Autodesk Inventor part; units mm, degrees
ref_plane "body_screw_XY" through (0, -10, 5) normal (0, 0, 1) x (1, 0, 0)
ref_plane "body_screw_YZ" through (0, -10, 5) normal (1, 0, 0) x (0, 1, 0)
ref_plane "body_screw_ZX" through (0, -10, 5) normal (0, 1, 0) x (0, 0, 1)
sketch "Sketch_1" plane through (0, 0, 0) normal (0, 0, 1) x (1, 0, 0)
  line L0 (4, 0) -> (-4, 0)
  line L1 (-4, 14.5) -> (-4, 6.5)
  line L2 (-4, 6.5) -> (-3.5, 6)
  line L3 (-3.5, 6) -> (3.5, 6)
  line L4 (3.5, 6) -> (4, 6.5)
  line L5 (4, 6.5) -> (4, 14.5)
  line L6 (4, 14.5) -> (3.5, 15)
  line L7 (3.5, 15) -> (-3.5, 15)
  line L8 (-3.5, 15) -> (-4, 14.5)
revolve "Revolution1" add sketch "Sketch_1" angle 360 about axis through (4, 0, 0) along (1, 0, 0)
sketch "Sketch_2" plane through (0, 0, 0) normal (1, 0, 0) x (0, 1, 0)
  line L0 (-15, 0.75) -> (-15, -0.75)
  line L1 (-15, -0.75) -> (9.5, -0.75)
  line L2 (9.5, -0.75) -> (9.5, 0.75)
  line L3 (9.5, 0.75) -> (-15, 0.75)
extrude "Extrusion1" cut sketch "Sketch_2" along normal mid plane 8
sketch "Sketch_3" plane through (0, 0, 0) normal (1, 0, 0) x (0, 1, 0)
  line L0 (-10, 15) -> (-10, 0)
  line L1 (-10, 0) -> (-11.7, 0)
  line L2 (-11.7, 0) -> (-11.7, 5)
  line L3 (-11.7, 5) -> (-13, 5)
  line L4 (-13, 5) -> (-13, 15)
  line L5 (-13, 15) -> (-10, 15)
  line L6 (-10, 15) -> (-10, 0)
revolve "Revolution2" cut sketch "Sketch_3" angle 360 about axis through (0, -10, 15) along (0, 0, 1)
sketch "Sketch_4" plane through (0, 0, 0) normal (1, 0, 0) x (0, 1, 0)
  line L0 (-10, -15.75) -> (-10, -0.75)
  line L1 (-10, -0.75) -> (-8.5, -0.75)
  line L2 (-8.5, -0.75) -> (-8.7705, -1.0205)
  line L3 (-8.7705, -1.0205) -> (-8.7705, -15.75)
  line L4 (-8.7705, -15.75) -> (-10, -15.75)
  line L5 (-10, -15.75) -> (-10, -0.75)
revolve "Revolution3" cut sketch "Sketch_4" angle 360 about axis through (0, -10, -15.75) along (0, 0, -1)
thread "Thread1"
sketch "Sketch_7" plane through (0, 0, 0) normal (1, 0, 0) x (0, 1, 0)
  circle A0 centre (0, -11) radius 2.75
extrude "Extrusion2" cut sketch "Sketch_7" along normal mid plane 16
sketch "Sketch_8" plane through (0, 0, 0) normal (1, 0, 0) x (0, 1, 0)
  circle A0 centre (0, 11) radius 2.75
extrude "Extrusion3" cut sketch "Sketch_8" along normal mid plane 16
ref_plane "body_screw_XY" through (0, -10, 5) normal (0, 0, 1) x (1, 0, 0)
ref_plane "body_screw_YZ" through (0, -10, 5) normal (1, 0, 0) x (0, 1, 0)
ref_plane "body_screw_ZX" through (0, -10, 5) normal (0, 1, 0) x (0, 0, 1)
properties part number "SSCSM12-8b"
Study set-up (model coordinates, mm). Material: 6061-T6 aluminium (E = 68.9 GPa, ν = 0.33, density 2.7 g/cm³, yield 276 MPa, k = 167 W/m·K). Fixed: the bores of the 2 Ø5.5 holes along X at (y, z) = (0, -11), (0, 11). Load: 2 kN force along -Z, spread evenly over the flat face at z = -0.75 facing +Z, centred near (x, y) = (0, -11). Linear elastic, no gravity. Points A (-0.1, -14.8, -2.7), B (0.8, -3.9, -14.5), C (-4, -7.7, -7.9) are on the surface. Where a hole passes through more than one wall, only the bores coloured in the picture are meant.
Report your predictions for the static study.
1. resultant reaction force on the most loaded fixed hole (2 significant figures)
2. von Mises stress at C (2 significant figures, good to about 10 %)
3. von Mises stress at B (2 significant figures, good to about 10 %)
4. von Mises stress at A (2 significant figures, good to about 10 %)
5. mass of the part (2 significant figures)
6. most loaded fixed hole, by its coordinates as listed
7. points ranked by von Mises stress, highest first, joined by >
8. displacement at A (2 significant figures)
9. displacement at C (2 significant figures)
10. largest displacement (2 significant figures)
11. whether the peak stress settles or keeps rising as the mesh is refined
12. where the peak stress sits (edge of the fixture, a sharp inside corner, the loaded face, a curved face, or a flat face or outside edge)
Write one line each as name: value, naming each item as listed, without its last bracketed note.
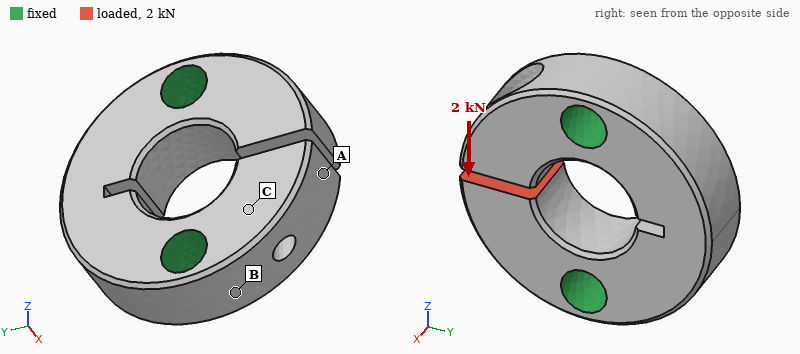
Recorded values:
resultant reaction force on the most loaded fixed hole: 2.1 kN
von Mises stress at C: 65 MPa
von Mises stress at B: 100 MPa
von Mises stress at A: 33 MPa
mass of the part: 11 g
most loaded fixed hole, by its coordinates as listed: (0, -11)
points ranked by von Mises stress, highest first, joined by >: B > C > A
displacement at A: 60 µm
displacement at C: 20 µm
largest displacement: 66 µm
whether the peak stress settles or keeps rising as the mesh is refined: keeps rising
where the peak stress sits: edge of the fixture
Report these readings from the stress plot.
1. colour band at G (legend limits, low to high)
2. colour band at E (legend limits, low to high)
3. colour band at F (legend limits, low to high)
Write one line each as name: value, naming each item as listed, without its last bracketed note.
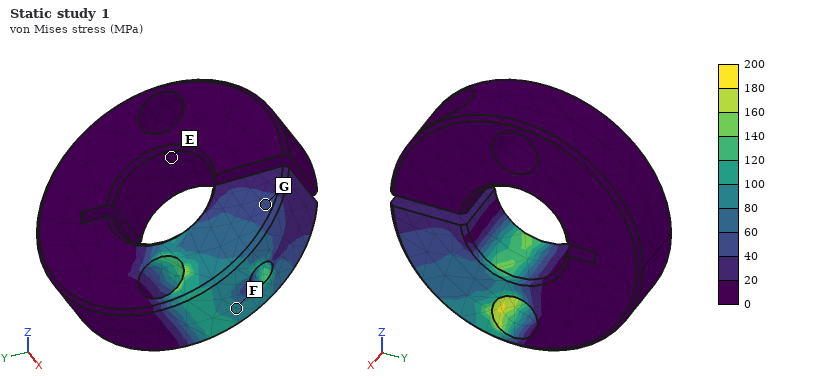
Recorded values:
colour band at G: 40 to 60 MPa
colour band at E: 0 to 20 MPa
colour band at F: 80 to 100 MPa
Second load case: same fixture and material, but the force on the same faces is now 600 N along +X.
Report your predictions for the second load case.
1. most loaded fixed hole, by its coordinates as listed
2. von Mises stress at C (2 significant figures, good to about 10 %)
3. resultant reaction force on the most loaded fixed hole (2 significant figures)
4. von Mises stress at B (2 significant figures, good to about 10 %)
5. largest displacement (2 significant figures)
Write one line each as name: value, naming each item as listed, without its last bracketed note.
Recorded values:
most loaded fixed hole, by its coordinates as listed: (0, -11)
von Mises stress at C: 45 MPa
resultant reaction force on the most loaded fixed hole: 600 N
von Mises stress at B: 30 MPa
largest displacement: 32 µm
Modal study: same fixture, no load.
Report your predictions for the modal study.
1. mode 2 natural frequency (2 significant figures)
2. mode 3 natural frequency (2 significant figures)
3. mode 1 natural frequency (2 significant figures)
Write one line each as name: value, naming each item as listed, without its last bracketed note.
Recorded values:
mode 2 natural frequency: 27 kHz
mode 3 natural frequency: 27 kHz
mode 1 natural frequency: 25 kHz
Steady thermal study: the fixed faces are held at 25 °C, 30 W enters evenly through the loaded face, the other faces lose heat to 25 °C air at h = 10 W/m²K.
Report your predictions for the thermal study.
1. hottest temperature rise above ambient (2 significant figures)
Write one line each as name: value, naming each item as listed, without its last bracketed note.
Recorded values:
hottest temperature rise above ambient: 40 K
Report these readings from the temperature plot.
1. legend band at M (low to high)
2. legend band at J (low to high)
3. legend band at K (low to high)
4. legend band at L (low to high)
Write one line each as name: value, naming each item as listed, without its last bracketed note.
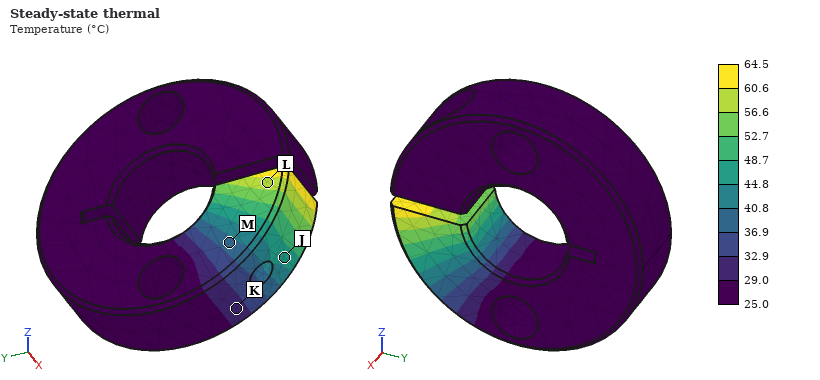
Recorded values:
legend band at M: 36.9 to 40.8 °C
legend band at J: 44.8 to 48.7 °C
legend band at K: 29.0 to 32.9 °C
legend band at L: 56.6 to 60.6 °C
